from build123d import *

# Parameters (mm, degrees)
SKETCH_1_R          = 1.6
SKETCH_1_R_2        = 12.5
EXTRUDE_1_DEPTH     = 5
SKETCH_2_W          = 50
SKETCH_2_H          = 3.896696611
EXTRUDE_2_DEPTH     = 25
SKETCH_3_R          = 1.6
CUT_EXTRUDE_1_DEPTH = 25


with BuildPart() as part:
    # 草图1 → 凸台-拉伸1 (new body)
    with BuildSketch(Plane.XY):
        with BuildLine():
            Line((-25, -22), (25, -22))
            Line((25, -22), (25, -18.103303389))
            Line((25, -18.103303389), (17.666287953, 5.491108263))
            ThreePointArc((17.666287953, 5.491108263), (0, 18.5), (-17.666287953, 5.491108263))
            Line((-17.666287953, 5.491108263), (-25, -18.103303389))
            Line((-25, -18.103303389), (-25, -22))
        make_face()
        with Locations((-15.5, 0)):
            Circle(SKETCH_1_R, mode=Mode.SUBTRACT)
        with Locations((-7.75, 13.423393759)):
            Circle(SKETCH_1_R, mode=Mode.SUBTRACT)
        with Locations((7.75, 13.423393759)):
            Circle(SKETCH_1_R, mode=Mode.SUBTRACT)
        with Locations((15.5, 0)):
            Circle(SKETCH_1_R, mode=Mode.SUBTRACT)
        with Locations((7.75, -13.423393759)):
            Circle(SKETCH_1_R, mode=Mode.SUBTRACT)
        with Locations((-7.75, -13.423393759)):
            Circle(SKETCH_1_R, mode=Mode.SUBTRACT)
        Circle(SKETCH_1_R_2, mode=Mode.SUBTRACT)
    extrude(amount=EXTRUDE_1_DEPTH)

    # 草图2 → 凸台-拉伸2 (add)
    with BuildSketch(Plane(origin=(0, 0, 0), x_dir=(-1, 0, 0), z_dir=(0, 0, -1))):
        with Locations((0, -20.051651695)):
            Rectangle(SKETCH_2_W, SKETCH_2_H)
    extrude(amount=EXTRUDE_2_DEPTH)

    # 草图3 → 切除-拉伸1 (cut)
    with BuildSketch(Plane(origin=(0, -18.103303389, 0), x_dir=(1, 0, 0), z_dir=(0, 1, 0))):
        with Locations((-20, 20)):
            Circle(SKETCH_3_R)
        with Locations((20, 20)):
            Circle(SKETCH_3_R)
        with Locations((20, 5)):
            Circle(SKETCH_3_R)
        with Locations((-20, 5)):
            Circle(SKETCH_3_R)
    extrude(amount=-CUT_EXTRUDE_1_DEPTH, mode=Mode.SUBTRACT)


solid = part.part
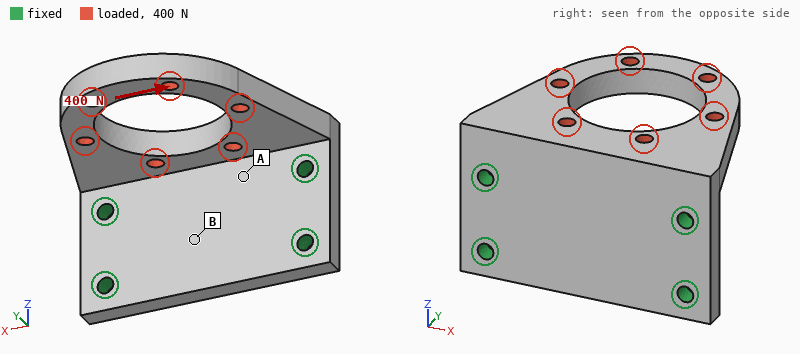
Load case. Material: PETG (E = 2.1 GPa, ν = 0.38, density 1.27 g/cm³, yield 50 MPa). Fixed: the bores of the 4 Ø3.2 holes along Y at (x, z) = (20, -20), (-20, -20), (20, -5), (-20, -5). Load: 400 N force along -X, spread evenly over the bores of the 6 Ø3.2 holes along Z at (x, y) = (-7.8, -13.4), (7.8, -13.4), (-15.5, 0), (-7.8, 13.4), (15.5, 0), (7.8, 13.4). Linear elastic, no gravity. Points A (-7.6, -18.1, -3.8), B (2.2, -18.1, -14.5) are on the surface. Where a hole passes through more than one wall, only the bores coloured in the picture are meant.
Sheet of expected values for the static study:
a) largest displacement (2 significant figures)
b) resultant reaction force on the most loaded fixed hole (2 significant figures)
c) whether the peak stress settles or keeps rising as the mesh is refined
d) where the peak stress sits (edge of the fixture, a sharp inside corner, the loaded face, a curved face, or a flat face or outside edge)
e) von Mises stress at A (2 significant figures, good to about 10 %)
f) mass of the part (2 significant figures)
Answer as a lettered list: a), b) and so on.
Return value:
a) 0.74 mm
b) 270 N
c) keeps rising
d) edge of the fixture
e) 5.7 MPa
f) 12 g
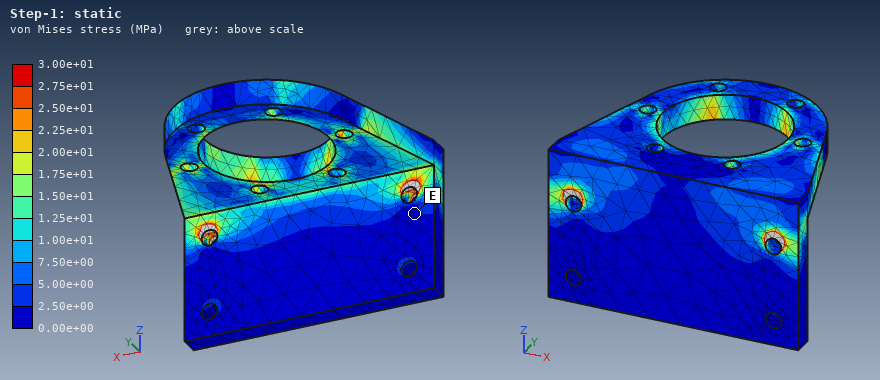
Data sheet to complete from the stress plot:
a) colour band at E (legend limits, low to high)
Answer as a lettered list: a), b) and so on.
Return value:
a) 0.00e+00 to 2.50e+00 MPa
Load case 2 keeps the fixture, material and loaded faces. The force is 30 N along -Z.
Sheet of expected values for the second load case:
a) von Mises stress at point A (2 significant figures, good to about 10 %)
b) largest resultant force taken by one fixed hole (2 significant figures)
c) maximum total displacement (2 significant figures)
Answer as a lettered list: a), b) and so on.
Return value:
a) 2.9 MPa
b) 13 N
c) 0.78 mm
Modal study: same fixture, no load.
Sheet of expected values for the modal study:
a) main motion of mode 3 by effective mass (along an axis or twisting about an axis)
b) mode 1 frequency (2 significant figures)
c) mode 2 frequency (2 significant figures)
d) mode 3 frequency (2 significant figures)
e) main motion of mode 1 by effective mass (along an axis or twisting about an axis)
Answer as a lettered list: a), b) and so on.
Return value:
a) along X
b) 640 Hz
c) 1600 Hz
d) 2400 Hz
e) along Z
